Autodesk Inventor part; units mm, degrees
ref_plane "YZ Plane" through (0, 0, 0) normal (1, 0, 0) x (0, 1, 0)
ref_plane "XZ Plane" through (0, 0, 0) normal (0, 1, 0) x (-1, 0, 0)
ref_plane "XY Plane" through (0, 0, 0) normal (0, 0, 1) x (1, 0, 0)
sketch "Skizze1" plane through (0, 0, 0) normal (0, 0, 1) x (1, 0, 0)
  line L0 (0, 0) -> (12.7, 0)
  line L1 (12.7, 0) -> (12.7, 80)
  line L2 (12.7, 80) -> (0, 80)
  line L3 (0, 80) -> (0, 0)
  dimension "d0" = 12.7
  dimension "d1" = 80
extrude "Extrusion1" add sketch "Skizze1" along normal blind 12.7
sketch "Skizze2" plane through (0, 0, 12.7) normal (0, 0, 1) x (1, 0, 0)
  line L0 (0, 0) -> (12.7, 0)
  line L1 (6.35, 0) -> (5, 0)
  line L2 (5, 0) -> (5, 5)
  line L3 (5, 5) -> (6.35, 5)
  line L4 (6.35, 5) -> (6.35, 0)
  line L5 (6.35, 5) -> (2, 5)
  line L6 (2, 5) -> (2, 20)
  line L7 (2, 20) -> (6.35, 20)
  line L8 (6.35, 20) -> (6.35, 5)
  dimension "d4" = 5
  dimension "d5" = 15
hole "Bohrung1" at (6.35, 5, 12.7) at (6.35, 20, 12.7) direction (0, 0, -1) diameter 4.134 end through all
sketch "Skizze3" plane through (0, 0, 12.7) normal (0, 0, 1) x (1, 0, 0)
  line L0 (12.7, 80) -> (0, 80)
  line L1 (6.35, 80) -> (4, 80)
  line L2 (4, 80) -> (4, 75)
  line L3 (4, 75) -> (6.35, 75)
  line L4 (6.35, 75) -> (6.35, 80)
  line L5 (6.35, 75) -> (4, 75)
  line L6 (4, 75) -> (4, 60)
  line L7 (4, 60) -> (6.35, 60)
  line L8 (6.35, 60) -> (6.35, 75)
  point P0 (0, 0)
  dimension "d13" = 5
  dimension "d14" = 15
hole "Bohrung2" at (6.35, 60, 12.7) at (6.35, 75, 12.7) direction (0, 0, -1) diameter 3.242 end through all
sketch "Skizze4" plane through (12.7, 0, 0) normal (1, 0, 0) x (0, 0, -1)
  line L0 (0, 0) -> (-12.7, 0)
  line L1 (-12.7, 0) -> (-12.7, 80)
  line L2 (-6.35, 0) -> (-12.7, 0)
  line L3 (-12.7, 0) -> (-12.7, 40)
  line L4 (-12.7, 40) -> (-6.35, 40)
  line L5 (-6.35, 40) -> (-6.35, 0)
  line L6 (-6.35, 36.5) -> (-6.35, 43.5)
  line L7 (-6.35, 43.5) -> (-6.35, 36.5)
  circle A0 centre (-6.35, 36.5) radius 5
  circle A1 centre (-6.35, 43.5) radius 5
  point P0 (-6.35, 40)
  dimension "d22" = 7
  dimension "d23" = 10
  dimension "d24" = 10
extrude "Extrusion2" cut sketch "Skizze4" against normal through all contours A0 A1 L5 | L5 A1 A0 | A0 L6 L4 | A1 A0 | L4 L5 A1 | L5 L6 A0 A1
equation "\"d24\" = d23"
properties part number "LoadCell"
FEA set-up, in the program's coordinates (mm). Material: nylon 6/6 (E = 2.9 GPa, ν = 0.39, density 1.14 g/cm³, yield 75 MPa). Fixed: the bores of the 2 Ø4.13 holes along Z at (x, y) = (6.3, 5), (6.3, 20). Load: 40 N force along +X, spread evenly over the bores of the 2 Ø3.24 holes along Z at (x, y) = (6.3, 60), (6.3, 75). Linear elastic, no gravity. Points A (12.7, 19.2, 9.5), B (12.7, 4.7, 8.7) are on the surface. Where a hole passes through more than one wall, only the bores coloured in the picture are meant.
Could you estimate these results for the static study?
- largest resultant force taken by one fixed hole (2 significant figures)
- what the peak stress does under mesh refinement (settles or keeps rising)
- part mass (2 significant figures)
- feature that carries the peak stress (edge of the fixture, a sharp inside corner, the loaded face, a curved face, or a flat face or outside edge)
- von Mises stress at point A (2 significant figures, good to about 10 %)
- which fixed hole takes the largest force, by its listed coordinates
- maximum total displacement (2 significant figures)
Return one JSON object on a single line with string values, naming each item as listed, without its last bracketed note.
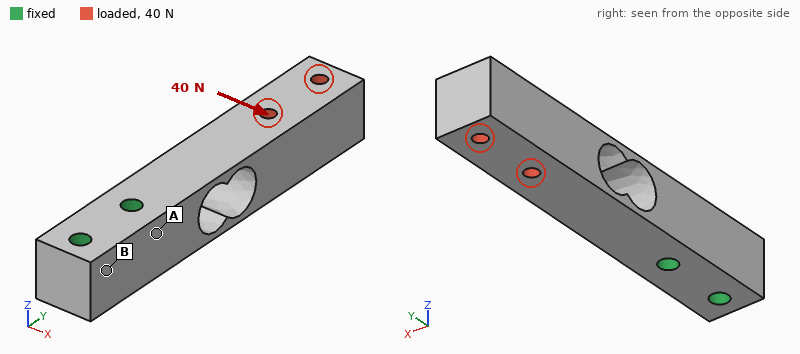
{"largest resultant force taken by one fixed hole": "100 N", "what the peak stress does under mesh refinement": "keeps rising", "part mass": "12 g", "feature that carries the peak stress": "a sharp inside corner", "von Mises stress at point A": "3.6 MPa", "which fixed hole takes the largest force, by its listed coordinates": "(6.3, 20)", "maximum total displacement": "0.85 mm"}
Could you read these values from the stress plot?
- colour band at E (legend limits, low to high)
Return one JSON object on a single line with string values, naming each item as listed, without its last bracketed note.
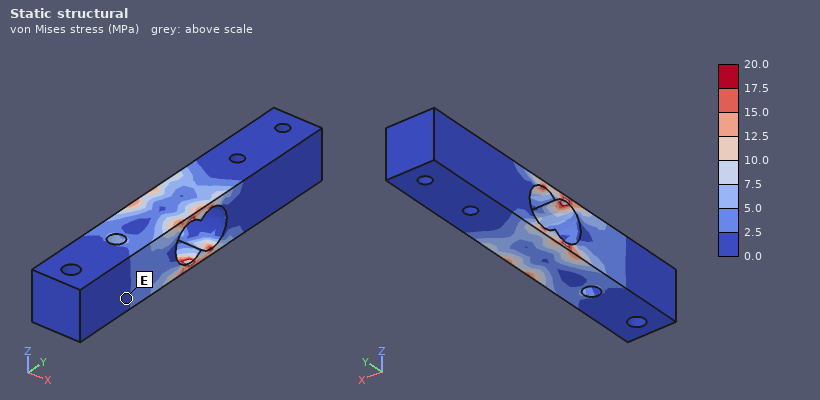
{"colour band at E": "0.0 to 2.5 MPa"}
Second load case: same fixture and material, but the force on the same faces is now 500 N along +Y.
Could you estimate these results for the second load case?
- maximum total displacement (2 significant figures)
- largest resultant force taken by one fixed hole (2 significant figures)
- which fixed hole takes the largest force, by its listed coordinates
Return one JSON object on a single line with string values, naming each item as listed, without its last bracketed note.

{"maximum total displacement": "0.13 mm", "largest resultant force taken by one fixed hole": "450 N", "which fixed hole takes the largest force, by its listed coordinates": "(6.3, 20)"}
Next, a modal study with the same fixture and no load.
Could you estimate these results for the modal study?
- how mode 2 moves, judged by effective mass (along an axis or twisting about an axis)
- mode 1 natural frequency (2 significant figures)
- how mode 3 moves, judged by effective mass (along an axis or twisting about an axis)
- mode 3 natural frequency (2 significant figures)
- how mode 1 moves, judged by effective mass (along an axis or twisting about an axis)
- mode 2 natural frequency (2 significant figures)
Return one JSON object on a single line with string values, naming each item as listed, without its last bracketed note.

{"how mode 2 moves, judged by effective mass": "along X", "mode 1 natural frequency": "540 Hz", "how mode 3 moves, judged by effective mass": "twisting about Y", "mode 3 natural frequency": "2200 Hz", "how mode 1 moves, judged by effective mass": "along Z", "mode 2 natural frequency": "580 Hz"}
